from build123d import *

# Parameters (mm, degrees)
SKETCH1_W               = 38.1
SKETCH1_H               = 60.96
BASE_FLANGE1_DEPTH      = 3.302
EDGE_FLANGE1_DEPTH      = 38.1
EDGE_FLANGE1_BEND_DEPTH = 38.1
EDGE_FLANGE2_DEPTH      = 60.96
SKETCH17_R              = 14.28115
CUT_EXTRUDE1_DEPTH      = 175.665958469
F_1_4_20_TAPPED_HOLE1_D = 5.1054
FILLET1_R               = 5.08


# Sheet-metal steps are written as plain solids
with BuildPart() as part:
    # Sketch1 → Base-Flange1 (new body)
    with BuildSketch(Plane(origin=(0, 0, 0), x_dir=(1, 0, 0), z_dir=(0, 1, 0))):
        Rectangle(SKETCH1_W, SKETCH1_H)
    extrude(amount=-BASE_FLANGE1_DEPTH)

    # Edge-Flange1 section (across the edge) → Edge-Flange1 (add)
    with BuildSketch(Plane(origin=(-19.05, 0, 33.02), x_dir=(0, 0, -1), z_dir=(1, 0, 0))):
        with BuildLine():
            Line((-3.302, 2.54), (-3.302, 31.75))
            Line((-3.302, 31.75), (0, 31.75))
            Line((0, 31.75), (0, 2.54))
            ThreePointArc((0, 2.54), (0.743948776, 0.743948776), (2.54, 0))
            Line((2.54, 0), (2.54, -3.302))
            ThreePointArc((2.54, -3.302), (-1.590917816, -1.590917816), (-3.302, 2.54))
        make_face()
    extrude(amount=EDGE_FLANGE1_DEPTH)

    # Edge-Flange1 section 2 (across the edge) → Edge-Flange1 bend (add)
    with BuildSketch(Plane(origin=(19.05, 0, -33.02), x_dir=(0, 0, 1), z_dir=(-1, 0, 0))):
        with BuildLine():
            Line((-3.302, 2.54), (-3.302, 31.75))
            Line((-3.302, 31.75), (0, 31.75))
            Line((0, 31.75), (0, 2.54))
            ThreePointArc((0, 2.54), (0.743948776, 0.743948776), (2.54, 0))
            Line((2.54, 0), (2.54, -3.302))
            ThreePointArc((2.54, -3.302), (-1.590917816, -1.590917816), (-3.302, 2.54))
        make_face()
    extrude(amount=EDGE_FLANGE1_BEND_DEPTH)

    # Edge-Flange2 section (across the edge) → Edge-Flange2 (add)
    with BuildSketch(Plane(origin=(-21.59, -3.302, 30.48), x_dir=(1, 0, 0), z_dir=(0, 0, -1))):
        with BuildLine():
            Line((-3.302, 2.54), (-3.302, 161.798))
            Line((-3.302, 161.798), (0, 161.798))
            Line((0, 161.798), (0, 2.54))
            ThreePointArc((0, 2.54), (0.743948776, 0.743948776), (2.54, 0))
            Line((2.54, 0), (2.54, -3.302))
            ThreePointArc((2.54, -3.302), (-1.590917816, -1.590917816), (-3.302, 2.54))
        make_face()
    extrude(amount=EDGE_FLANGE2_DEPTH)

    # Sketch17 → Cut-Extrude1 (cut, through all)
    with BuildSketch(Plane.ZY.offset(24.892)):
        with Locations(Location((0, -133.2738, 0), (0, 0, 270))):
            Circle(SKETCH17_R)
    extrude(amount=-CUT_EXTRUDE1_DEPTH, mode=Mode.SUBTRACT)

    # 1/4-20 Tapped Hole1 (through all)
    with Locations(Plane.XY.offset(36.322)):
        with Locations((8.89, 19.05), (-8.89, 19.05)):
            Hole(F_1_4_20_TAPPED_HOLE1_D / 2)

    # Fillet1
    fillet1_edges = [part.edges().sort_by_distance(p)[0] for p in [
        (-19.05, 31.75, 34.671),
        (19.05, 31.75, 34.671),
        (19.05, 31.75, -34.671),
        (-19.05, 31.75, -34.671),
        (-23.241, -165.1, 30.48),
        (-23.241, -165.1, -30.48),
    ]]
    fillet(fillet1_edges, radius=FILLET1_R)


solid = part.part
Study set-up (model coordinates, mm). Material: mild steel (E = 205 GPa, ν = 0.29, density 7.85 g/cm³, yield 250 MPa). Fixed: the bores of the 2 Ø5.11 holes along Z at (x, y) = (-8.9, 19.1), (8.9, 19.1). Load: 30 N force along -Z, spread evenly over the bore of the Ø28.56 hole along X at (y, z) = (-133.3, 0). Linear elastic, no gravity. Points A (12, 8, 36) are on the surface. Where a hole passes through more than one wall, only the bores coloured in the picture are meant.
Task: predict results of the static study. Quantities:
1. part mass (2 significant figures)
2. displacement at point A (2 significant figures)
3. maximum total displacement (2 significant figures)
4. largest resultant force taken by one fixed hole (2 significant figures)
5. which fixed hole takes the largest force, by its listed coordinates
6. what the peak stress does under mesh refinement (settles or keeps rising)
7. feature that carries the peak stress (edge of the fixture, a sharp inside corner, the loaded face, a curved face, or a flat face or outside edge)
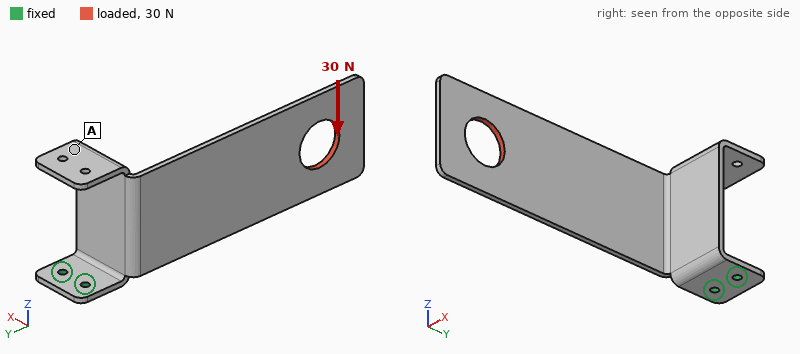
370 g
0.37 mm
1.1 mm
50 N
(-8.9, 19.1)
keeps rising
a sharp inside corner
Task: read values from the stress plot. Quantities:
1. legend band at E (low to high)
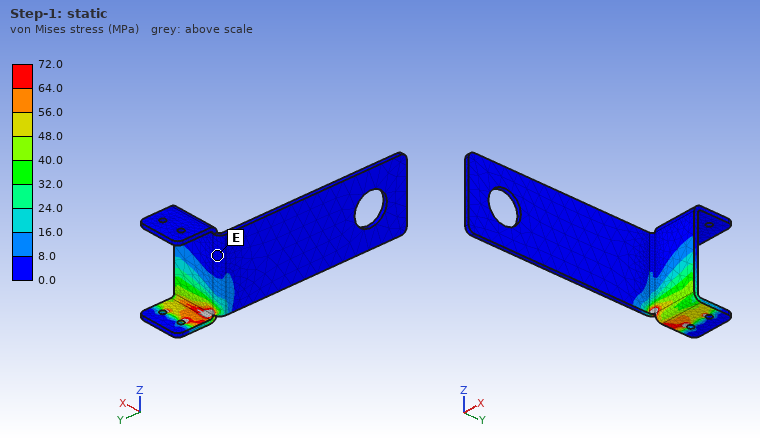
0.0 to 8.0 MPa
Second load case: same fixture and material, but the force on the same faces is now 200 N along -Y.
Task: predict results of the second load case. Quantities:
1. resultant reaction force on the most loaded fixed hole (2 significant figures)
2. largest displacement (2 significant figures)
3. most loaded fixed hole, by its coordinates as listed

320 N
1.8 mm
(-8.9, 19.1)
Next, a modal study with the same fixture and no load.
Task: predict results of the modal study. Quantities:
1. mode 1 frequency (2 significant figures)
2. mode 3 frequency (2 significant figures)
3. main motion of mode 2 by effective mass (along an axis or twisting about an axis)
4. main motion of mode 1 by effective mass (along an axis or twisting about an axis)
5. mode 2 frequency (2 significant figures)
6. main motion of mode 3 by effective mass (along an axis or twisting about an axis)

74 Hz
410 Hz
along X
along Z
92 Hz
along X
